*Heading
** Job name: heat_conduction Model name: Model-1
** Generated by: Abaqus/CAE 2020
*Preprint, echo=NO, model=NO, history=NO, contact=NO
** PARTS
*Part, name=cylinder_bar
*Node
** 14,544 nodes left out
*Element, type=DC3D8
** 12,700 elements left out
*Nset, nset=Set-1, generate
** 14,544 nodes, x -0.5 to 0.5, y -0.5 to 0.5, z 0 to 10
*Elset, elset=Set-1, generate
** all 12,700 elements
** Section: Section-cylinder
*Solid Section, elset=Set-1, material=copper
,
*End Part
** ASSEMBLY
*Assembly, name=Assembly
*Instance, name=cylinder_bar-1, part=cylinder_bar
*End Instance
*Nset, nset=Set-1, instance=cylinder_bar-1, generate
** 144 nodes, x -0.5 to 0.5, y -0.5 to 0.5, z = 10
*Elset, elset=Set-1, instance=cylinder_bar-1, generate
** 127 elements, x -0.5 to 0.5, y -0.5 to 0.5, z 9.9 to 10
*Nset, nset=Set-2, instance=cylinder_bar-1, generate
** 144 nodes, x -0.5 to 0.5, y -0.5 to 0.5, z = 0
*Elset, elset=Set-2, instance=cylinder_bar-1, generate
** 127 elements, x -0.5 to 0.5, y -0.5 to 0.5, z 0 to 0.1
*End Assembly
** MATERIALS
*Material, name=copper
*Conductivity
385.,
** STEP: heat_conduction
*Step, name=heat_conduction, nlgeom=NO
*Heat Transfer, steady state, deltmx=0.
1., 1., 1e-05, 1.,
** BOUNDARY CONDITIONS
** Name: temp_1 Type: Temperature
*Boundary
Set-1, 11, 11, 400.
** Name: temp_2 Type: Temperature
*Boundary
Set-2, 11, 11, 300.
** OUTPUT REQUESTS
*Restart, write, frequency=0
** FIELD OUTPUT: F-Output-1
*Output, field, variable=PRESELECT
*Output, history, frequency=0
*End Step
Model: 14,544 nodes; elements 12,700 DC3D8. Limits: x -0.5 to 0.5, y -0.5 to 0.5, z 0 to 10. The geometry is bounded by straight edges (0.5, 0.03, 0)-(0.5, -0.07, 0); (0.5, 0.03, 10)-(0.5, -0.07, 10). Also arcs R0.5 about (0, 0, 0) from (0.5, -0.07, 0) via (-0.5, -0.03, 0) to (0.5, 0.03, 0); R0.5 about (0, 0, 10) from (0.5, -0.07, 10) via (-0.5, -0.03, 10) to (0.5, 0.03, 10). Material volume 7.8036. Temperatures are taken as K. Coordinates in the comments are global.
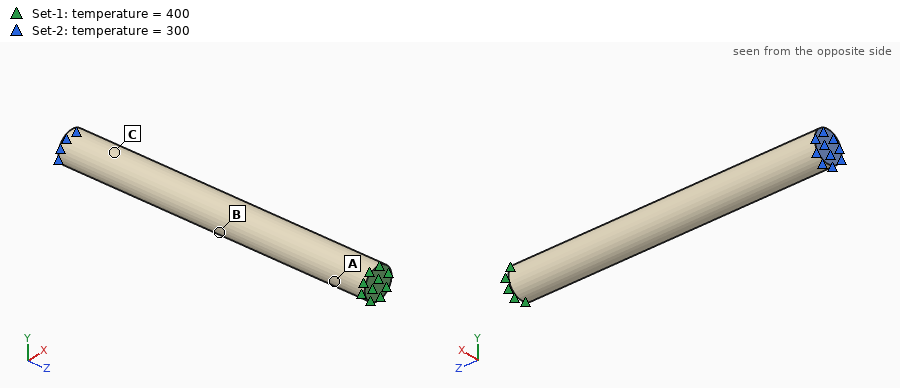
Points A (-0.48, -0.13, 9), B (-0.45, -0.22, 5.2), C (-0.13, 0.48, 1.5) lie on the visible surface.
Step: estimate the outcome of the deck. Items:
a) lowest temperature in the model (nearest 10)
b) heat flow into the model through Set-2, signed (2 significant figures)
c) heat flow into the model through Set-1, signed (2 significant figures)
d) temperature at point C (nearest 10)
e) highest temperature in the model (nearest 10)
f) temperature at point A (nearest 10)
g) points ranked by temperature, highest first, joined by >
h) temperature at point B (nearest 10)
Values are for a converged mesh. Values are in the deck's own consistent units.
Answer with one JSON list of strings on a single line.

["300 K", "-3000", "3000", "320 K", "400 K", "390 K", "A > B > C", "350 K"]
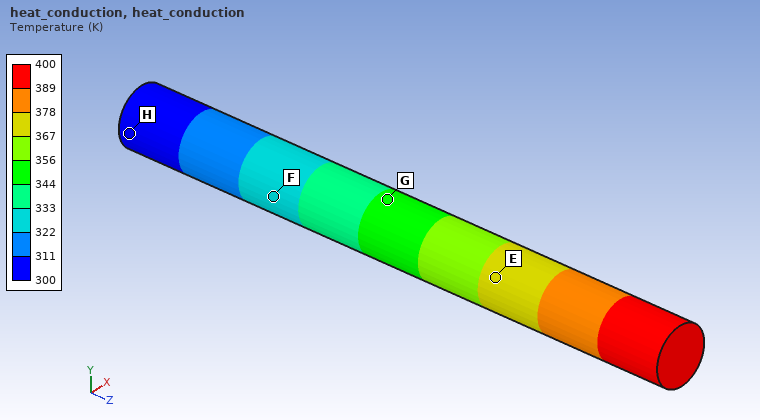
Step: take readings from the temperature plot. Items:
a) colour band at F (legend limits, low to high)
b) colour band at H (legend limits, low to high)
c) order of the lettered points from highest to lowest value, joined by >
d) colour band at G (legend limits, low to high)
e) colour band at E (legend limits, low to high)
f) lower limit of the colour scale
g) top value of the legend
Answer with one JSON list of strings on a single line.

["322 to 333 K", "300 to 311 K", "E > G > F > H", "344 to 356 K", "367 to 378 K", "300 K", "400 K"]
